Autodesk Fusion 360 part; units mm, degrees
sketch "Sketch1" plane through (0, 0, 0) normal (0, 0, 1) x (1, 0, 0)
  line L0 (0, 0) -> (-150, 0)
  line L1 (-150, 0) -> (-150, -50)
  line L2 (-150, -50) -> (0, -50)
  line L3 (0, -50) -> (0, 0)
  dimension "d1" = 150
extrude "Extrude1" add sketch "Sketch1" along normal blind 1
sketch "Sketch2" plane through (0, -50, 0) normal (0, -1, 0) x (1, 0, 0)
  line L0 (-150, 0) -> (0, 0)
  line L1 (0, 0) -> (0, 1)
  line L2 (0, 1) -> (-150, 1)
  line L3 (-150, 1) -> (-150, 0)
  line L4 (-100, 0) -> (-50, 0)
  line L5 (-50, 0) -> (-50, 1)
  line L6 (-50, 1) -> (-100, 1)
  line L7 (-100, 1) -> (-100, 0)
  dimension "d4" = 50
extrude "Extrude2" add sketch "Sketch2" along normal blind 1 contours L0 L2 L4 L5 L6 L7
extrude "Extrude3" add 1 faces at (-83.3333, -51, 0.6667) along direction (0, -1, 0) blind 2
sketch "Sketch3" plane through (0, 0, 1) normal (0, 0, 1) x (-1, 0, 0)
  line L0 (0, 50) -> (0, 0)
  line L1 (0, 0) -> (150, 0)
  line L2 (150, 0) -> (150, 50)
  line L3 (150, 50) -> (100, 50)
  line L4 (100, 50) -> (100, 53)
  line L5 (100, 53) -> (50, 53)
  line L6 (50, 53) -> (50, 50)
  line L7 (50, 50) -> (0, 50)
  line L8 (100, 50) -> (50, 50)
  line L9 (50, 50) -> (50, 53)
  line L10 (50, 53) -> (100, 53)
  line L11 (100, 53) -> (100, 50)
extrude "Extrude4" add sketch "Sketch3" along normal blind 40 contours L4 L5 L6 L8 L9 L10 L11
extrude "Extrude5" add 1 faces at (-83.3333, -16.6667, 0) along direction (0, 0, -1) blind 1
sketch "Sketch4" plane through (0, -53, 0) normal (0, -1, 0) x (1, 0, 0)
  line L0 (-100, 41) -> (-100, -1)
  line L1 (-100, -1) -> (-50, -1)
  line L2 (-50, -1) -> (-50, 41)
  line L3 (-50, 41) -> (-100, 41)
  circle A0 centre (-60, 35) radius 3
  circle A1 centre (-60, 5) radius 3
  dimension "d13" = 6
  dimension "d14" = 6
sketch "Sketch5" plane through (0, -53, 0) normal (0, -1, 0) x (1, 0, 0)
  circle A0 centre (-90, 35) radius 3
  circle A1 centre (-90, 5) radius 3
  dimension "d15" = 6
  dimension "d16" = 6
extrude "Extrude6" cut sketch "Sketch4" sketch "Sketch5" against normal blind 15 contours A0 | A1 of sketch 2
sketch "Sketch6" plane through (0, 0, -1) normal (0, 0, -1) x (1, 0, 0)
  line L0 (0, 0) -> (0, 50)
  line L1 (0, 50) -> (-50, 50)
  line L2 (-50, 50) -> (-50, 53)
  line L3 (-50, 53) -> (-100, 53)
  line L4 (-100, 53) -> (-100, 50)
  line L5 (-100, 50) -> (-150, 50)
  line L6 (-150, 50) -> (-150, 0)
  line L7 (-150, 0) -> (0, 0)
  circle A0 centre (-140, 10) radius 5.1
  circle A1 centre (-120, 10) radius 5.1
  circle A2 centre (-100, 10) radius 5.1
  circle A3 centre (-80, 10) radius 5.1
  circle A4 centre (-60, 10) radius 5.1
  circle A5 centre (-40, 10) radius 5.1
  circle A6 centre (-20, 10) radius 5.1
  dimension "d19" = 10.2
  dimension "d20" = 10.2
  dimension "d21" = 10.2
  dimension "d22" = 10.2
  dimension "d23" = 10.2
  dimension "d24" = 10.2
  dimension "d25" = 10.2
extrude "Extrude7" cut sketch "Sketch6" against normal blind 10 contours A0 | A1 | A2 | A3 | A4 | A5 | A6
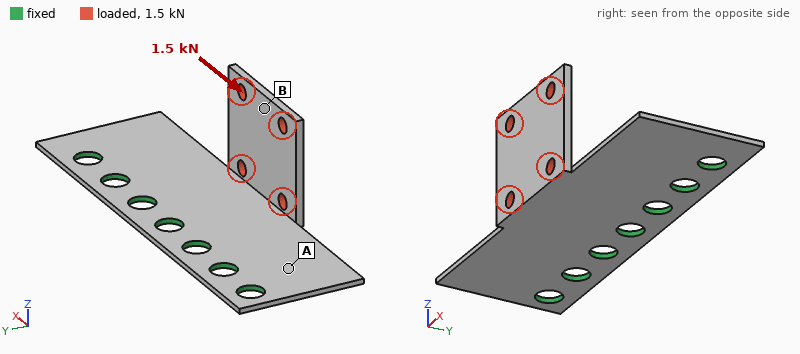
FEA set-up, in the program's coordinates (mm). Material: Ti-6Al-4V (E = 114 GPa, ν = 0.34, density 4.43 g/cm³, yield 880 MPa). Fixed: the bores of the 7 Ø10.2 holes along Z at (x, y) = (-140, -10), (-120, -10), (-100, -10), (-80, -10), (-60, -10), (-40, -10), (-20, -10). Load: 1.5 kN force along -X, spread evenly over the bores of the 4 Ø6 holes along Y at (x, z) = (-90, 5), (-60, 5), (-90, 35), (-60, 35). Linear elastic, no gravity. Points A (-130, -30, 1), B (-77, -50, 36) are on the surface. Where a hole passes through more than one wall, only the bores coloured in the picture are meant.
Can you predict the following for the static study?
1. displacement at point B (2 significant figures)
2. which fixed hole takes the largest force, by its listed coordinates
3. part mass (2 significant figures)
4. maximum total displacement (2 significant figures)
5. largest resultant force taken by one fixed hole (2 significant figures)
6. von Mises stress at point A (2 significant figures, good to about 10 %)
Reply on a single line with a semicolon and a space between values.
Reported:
1.4 mm; (-20, -10); 88 g; 1.9 mm; 430 N; 110 MPa
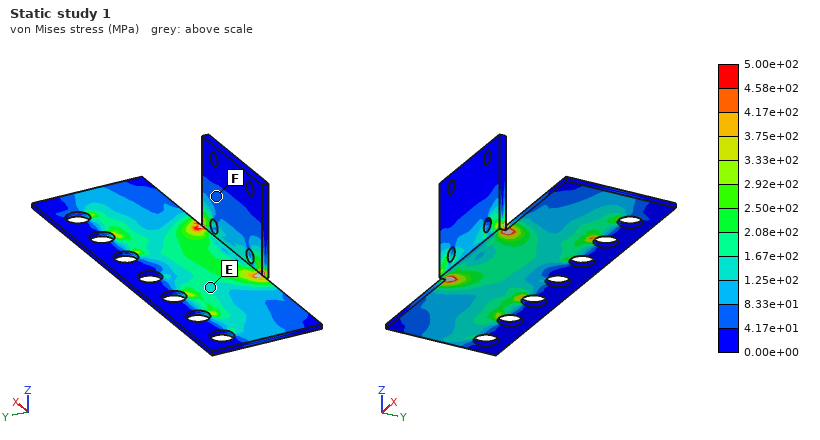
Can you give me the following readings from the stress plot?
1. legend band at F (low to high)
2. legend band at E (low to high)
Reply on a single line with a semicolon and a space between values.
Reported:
4.17e+01 to 8.33e+01 MPa; 1.25e+02 to 1.67e+02 MPa
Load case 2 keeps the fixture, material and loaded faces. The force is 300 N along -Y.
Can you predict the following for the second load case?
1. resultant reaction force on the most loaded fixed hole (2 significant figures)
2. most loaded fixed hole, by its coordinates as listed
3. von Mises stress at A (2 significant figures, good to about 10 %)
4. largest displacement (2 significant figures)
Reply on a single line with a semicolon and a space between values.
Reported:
120 N; (-80, -10); 39 MPa; 1.5 mm
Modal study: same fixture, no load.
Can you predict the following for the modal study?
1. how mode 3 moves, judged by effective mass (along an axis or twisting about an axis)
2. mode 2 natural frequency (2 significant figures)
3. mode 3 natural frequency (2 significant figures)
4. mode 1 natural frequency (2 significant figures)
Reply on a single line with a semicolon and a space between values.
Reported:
along Z; 890 Hz; 1100 Hz; 450 Hz
